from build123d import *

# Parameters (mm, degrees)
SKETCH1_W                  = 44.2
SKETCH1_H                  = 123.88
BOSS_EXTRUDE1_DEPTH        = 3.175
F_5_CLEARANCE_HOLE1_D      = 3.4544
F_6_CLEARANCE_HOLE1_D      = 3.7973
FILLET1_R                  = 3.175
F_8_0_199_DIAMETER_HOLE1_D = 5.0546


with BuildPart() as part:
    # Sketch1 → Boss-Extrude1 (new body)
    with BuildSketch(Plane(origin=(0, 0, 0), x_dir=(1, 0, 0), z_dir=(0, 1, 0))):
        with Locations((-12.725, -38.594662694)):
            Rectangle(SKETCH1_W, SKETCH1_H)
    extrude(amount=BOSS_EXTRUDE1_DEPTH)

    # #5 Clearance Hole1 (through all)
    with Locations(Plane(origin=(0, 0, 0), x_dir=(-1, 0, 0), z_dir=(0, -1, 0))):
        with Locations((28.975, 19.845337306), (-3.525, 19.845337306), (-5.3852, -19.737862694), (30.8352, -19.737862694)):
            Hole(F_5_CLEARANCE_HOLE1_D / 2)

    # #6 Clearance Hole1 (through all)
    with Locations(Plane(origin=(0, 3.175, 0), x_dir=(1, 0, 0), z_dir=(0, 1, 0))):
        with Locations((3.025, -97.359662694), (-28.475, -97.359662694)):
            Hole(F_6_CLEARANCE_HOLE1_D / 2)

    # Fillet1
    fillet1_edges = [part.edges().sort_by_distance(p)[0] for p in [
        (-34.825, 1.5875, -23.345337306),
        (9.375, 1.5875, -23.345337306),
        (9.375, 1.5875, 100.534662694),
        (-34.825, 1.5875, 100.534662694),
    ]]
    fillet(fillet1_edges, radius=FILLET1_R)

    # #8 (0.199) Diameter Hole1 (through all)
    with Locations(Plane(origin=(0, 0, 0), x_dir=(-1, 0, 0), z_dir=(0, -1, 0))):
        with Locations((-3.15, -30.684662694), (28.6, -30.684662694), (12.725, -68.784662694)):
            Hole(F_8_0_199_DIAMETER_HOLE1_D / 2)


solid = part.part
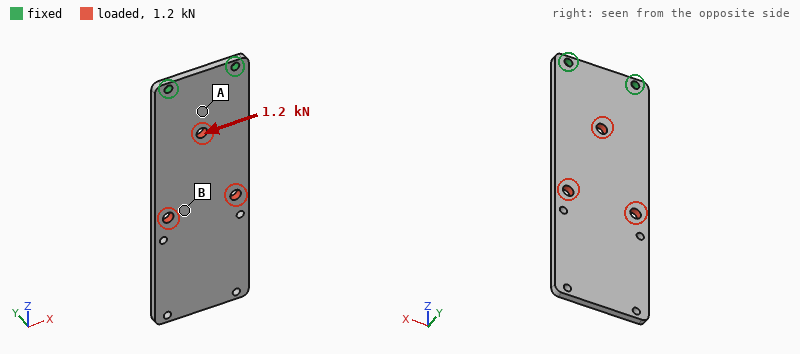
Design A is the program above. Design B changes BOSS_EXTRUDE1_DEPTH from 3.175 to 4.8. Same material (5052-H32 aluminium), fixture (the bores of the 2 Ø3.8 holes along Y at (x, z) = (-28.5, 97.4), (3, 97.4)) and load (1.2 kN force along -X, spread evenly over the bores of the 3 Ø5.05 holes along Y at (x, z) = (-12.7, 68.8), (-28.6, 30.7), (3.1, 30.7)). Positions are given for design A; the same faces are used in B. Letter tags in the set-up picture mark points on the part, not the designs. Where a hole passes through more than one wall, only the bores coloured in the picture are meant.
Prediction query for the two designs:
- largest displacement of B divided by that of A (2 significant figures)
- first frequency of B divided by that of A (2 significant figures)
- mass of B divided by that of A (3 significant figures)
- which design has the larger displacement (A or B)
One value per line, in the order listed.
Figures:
0.66
1.5
1.51
A
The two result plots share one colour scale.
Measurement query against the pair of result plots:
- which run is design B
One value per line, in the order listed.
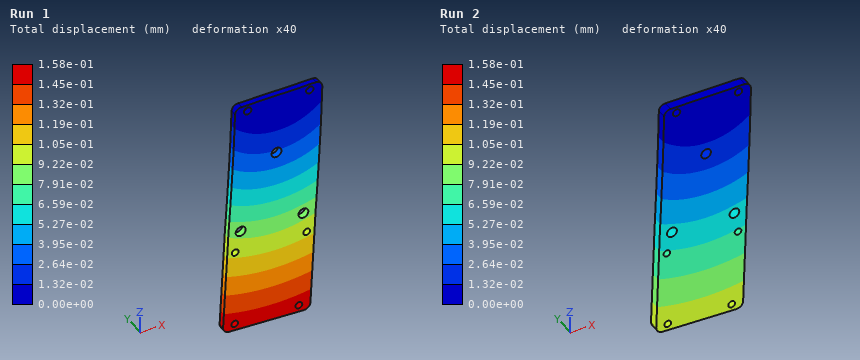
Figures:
Run 2
